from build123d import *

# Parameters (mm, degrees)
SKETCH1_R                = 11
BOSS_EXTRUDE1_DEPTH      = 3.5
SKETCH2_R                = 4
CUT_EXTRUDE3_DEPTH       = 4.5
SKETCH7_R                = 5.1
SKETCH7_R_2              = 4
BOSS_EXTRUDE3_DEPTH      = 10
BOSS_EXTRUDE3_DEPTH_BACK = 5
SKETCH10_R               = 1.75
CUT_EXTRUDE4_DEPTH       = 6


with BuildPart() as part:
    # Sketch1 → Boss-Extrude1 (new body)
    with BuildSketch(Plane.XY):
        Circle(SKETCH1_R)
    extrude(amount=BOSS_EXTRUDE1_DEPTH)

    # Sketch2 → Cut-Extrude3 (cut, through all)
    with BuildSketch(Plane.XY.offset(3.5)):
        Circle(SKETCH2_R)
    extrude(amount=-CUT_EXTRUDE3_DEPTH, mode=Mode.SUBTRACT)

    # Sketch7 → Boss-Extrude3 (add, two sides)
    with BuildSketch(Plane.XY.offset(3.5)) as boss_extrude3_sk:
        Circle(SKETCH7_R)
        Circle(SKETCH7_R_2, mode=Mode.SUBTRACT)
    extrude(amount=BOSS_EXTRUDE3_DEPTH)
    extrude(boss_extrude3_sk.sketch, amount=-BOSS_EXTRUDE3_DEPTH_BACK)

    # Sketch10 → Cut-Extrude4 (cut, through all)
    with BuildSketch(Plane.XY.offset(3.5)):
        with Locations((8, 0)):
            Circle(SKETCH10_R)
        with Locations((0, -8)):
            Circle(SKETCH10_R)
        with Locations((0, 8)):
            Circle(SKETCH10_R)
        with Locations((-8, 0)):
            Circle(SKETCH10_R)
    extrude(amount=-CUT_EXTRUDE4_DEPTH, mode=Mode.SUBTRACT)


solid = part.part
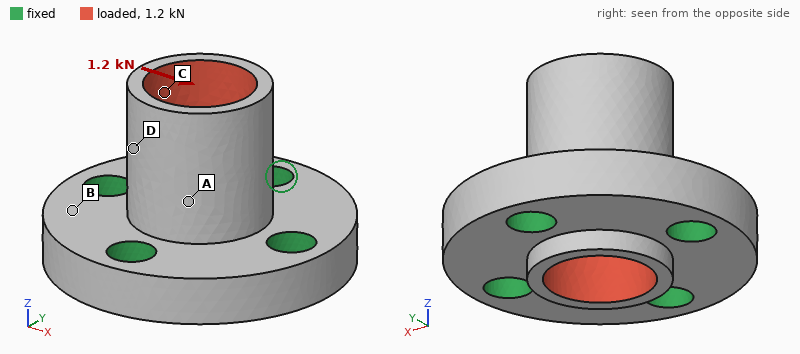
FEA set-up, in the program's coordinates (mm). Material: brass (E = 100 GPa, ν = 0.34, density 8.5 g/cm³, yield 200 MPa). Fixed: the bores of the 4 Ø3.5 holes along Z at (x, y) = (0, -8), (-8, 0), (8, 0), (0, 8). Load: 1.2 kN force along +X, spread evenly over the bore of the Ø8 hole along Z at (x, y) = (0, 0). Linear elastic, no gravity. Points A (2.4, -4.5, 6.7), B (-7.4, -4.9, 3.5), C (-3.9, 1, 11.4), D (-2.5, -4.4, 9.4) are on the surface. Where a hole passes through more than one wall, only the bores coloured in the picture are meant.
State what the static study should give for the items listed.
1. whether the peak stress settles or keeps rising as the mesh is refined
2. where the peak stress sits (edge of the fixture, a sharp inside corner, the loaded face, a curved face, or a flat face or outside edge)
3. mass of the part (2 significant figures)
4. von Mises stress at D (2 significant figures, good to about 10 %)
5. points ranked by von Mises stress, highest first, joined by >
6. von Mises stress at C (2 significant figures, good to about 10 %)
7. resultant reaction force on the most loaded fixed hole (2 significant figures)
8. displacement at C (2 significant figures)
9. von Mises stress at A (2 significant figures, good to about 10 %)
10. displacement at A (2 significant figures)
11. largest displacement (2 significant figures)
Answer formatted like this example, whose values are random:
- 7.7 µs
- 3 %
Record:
- keeps rising
- a sharp inside corner
- 12 g
- 30 MPa
- A > D > C > B
- 17 MPa
- 500 N
- 12 µm
- 45 MPa
- 5.9 µm
- 14 µm
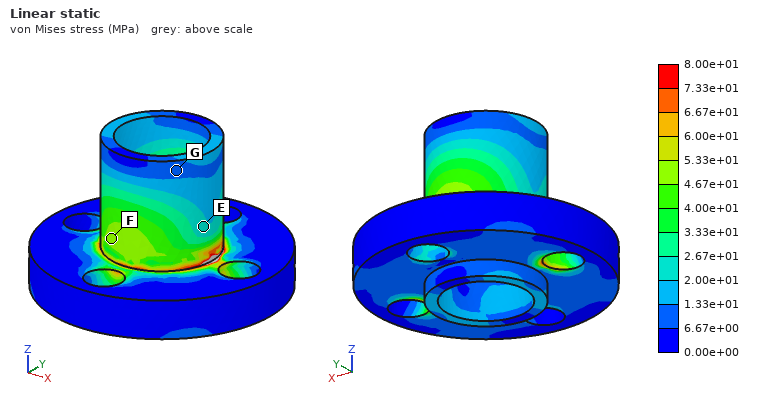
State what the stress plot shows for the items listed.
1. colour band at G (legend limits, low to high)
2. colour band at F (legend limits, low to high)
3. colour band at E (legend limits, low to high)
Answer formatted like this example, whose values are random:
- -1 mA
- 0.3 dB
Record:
- 6.67e+00 to 1.33e+01 MPa
- 4.67e+01 to 5.33e+01 MPa
- 2.00e+01 to 2.67e+01 MPa
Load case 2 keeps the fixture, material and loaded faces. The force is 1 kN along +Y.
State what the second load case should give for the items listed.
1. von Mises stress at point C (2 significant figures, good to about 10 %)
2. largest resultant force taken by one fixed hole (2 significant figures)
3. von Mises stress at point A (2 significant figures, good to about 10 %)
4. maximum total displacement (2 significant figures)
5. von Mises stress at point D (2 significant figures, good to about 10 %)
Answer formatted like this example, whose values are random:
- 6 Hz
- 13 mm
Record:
- 17 MPa
- 420 N
- 24 MPa
- 12 µm
- 18 MPa
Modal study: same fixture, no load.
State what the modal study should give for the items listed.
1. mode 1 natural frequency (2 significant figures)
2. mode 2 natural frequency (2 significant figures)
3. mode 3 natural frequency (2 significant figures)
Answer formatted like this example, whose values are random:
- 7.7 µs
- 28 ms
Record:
- 27 kHz
- 27 kHz
- 28 kHz
